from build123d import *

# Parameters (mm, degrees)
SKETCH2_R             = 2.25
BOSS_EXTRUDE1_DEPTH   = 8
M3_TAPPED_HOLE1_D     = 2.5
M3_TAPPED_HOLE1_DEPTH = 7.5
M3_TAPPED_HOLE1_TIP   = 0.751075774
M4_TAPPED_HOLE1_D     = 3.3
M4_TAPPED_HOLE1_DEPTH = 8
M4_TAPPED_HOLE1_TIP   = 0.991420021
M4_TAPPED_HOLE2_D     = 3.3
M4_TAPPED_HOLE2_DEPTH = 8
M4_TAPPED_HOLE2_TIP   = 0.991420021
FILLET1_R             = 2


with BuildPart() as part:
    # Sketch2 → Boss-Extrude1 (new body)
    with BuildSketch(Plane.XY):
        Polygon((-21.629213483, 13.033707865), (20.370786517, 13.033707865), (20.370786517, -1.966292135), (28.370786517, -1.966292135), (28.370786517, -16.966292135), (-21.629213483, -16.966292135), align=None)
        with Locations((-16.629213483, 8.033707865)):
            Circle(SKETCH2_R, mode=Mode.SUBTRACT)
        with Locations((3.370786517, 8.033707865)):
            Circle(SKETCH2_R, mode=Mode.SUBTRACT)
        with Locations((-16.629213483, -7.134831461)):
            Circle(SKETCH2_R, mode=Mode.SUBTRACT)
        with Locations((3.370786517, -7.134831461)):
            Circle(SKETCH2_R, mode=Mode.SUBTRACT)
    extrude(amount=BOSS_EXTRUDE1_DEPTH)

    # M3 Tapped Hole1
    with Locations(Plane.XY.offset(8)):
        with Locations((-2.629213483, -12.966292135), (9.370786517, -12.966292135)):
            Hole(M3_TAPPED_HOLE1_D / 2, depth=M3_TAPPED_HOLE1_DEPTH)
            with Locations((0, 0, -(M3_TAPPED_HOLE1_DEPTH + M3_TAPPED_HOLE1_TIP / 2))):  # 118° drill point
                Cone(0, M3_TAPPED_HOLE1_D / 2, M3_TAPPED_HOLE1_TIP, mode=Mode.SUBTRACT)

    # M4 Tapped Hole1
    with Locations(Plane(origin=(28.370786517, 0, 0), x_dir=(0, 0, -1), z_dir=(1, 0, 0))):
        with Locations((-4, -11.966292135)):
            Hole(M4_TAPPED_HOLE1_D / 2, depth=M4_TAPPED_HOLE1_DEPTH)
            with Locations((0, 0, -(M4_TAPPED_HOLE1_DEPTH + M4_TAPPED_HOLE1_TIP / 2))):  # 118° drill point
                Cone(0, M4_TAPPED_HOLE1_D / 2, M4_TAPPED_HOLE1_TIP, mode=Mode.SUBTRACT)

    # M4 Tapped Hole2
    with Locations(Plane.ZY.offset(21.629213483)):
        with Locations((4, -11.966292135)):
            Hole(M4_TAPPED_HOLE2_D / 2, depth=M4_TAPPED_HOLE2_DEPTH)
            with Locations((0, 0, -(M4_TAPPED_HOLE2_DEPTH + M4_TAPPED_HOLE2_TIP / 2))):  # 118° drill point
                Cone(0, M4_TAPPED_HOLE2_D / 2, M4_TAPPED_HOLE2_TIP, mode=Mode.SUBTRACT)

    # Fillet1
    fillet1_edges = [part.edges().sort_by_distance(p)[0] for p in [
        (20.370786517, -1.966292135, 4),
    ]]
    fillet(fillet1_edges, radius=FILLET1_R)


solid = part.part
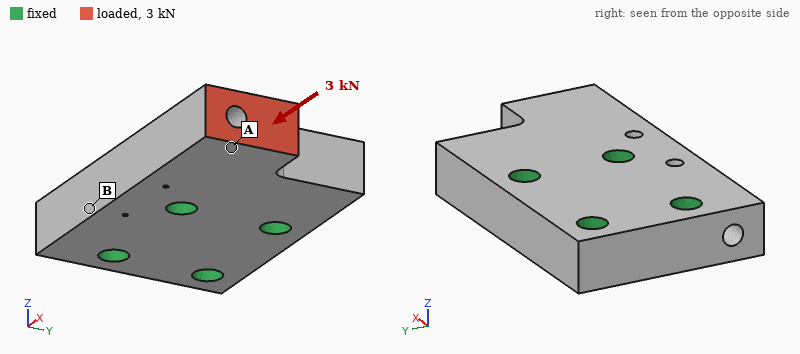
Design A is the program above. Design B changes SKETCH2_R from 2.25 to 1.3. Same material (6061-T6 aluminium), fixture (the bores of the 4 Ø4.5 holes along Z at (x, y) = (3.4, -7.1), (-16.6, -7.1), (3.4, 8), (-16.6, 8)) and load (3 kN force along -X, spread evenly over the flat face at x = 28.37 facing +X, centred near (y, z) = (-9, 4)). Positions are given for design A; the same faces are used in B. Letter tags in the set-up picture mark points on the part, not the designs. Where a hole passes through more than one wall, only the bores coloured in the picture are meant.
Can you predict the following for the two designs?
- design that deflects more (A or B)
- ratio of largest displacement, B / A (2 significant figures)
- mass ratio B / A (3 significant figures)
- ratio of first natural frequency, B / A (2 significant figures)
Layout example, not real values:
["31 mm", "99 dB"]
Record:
["B", "1.1", "1.03", "0.90"]
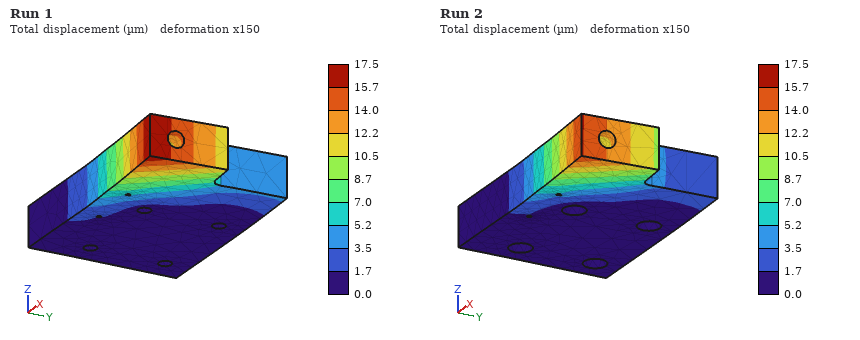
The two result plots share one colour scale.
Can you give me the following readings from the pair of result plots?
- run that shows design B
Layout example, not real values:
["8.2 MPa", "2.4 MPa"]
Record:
["Run 1"]
